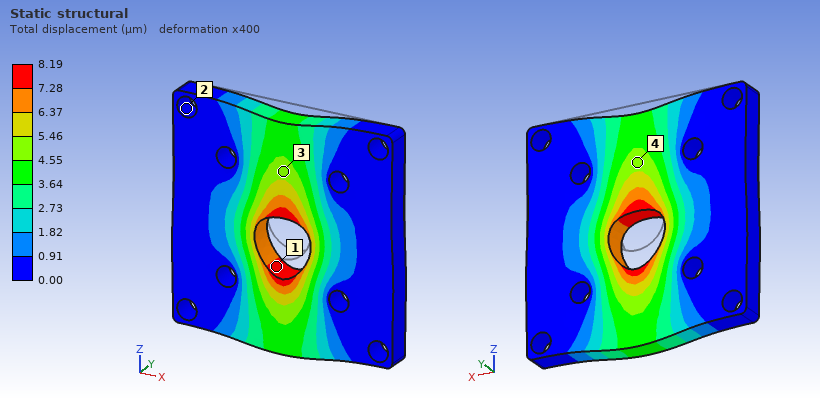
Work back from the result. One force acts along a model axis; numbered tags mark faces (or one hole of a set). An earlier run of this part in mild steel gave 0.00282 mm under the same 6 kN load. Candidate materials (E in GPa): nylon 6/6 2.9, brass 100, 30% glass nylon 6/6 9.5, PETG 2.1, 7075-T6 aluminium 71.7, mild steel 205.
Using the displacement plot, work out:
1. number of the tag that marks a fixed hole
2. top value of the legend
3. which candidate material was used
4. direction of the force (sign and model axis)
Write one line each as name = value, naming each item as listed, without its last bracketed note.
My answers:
number of the tag that marks a fixed hole = 2
top value of the legend = 8.19 µm
which candidate material was used = 7075-T6 aluminium
direction of the force = -Z
